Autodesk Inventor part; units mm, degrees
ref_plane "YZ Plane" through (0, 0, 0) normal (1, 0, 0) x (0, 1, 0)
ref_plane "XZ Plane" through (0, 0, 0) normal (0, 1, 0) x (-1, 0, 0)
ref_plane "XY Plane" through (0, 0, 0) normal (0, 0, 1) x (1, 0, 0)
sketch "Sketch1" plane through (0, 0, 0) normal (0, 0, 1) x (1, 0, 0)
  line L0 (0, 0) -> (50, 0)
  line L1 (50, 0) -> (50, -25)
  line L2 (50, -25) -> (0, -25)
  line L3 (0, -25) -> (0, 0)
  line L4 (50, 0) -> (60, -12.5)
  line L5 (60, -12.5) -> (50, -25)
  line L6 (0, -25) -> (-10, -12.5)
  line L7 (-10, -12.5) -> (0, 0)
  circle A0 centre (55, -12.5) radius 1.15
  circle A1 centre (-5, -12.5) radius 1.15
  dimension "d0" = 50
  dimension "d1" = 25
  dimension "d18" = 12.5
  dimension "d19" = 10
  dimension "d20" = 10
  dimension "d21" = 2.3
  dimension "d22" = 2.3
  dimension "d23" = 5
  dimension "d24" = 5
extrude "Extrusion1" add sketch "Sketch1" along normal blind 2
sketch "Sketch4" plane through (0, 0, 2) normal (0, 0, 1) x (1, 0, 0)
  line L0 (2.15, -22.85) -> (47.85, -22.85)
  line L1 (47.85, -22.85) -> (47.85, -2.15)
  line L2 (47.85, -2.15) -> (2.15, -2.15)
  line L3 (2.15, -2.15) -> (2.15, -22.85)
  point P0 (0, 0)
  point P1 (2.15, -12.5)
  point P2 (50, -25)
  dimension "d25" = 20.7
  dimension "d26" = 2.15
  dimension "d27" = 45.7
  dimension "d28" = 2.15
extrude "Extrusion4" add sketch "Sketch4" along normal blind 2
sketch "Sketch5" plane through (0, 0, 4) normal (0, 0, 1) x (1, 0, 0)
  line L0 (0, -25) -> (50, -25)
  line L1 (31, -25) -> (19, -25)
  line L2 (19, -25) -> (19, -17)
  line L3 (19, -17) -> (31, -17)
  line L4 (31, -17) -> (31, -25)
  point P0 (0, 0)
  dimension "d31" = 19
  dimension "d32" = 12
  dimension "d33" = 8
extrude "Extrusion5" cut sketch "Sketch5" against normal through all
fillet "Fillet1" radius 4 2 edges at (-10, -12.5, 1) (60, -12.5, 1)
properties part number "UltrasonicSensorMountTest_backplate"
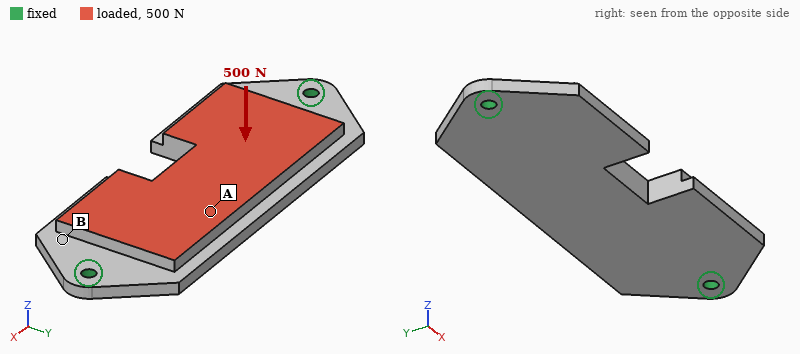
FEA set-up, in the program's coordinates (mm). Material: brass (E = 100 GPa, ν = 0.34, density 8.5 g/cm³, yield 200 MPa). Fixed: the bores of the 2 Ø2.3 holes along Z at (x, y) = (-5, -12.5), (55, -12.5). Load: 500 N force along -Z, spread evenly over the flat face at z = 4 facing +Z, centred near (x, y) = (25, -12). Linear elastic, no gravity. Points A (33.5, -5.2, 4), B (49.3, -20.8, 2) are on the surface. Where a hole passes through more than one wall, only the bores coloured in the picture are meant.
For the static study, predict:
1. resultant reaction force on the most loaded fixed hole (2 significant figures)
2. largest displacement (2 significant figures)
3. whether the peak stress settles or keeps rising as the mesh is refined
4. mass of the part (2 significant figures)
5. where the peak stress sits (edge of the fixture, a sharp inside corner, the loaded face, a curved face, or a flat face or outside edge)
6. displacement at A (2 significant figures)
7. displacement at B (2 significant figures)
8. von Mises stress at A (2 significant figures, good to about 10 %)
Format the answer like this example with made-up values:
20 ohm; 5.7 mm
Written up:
570 N; 0.10 mm; keeps rising; 39 g; edge of the fixture; 0.087 mm; 0.021 mm; 54 MPa
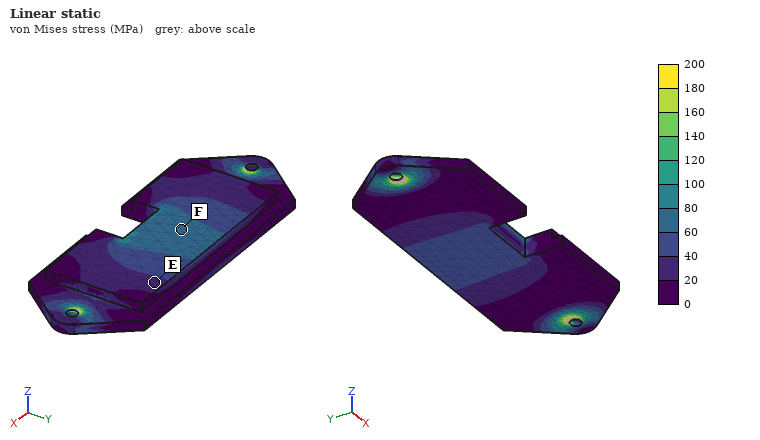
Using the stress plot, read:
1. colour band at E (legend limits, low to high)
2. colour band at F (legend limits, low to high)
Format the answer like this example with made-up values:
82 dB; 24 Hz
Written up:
20 to 40 MPa; 60 to 80 MPa
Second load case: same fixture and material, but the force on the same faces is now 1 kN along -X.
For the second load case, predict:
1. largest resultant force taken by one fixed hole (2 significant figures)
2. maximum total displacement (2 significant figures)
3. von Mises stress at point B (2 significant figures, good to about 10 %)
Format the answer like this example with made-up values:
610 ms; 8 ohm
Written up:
500 N; 4.1 µm; 13 MPa
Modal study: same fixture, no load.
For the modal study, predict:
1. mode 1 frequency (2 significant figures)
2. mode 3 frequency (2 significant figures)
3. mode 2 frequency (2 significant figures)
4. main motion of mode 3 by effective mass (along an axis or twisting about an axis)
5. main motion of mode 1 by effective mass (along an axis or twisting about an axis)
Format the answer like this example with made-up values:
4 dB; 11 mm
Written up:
2200 Hz; 5800 Hz; 2700 Hz; twisting about Y; along Z
